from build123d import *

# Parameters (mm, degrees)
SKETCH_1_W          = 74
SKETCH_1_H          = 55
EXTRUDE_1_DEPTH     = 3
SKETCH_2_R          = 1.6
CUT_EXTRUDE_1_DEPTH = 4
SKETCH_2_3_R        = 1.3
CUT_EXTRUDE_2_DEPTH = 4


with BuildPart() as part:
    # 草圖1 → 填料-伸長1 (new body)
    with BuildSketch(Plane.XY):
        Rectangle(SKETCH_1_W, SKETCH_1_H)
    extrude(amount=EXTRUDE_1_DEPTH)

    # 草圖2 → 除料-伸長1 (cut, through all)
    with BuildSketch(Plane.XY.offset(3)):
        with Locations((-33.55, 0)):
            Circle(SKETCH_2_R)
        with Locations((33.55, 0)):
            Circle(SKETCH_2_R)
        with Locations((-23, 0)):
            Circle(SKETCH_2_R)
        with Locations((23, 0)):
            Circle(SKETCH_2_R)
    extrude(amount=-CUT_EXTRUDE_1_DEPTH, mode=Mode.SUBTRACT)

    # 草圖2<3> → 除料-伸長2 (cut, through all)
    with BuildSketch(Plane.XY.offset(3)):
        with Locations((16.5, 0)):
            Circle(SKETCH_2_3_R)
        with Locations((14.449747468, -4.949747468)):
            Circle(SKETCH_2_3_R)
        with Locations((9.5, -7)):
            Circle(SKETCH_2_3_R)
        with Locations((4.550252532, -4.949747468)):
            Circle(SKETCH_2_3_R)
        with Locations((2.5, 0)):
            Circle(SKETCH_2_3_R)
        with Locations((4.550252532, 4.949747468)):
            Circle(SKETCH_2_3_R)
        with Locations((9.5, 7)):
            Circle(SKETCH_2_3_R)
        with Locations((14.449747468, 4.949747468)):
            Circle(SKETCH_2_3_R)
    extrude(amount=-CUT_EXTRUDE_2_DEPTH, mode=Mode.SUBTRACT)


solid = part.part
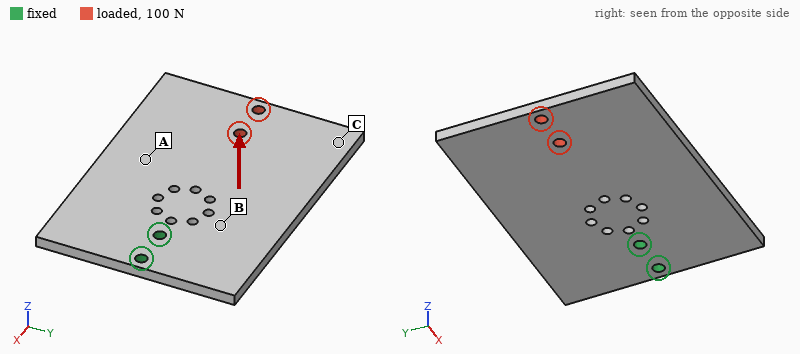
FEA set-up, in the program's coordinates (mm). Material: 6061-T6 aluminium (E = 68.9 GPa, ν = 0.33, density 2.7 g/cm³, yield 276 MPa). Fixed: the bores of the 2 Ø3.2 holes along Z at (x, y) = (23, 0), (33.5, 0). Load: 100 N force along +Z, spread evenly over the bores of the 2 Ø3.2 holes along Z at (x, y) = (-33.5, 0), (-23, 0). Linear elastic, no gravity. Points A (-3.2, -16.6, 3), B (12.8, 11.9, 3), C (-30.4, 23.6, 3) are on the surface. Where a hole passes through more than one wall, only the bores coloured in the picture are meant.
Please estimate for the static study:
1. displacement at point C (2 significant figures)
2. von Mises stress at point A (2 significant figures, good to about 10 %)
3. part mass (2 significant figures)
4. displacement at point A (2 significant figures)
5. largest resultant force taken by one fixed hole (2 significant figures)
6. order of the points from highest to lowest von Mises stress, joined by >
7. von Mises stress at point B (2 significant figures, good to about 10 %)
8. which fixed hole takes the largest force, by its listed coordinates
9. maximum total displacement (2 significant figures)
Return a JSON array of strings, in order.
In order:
["0.72 mm", "31 MPa", "32 g", "0.25 mm", "360 N", "B > A > C", "55 MPa", "(23, 0)", "0.88 mm"]
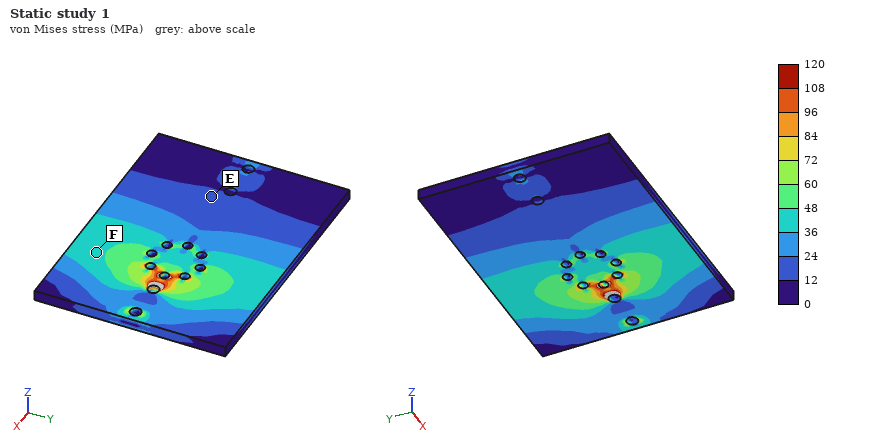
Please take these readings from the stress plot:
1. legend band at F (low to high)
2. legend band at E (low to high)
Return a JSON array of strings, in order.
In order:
["36 to 48 MPa", "12 to 24 MPa"]
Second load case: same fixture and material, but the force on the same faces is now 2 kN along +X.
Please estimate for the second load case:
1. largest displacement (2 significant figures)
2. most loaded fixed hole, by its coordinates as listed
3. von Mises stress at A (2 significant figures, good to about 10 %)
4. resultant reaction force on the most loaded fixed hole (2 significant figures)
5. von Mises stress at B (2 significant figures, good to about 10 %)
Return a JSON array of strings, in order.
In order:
["26 µm", "(23, 0)", "12 MPa", "1.4 kN", "18 MPa"]
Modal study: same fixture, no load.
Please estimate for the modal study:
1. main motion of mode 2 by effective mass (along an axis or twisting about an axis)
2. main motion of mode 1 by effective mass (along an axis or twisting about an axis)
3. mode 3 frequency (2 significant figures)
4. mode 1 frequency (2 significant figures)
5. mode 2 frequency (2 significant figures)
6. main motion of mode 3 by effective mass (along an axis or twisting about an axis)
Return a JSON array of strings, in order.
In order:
["twisting about X", "along Z", "3000 Hz", "590 Hz", "1200 Hz", "along Z"]
